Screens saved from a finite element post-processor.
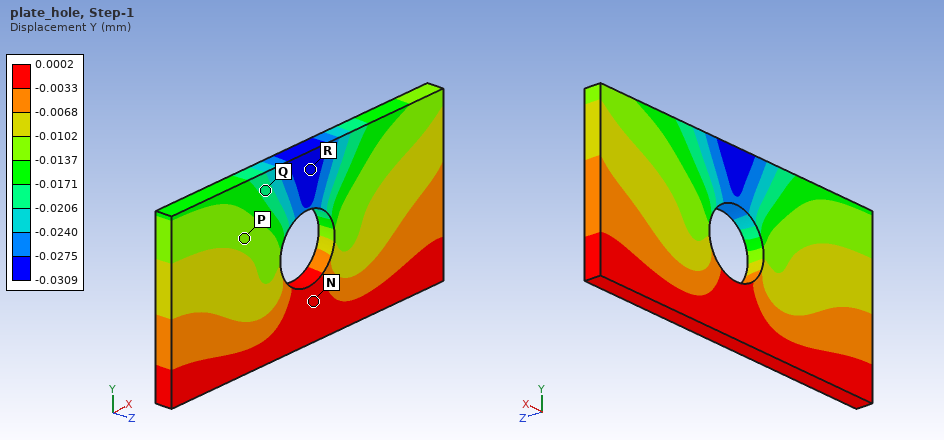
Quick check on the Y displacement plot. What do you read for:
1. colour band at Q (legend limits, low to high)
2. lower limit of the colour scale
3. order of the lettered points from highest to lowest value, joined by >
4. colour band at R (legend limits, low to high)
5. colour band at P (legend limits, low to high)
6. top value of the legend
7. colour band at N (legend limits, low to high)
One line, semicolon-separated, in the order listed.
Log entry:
-0.0206 to -0.0171 mm; -0.0309 mm; N > P > Q > R; -0.0309 to -0.0275 mm; -0.0137 to -0.0102 mm; 0.0002 mm; -0.0033 to 0.0002 mm
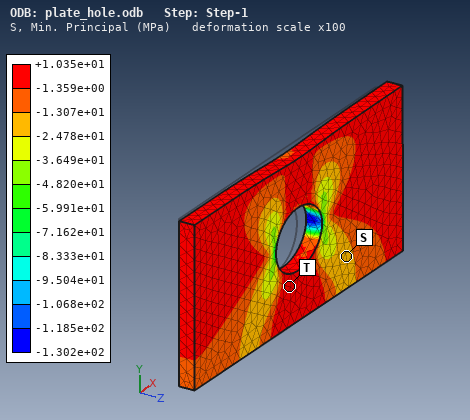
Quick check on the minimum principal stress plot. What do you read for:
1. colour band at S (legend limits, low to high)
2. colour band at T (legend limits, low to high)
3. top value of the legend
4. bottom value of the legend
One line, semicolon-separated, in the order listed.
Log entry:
-2.478e+01 to -1.307e+01 MPa; -1.359e+00 to +1.035e+01 MPa; +1.035e+01 MPa; -1.302e+02 MPa
